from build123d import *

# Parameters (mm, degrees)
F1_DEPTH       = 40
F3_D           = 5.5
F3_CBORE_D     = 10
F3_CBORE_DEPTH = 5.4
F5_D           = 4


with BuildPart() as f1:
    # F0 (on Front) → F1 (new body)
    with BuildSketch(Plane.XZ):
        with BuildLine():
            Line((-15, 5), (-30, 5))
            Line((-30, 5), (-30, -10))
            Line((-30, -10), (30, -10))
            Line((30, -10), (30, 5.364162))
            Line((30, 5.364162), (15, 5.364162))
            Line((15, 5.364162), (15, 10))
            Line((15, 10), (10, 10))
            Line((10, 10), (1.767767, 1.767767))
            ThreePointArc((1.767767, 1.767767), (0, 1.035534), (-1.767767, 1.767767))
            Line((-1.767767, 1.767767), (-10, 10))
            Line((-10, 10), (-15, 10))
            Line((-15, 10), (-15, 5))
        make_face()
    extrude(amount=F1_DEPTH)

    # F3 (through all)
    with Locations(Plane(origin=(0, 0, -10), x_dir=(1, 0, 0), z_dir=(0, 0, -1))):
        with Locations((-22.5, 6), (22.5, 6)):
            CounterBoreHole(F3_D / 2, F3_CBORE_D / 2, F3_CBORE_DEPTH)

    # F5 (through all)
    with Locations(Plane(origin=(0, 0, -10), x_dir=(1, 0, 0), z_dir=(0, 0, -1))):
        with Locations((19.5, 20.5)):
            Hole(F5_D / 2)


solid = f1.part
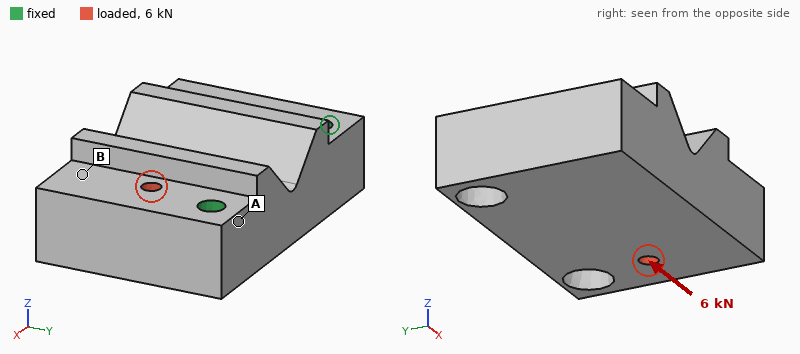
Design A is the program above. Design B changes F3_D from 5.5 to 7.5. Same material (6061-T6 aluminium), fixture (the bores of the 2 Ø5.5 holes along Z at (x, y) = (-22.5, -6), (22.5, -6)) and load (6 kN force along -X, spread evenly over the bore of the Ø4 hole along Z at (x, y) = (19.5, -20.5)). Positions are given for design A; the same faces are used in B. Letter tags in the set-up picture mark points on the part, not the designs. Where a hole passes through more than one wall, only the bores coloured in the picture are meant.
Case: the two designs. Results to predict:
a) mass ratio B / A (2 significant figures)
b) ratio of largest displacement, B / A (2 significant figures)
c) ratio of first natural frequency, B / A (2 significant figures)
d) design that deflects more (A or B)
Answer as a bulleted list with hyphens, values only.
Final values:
- 0.99
- 0.90
- 1.2
- A
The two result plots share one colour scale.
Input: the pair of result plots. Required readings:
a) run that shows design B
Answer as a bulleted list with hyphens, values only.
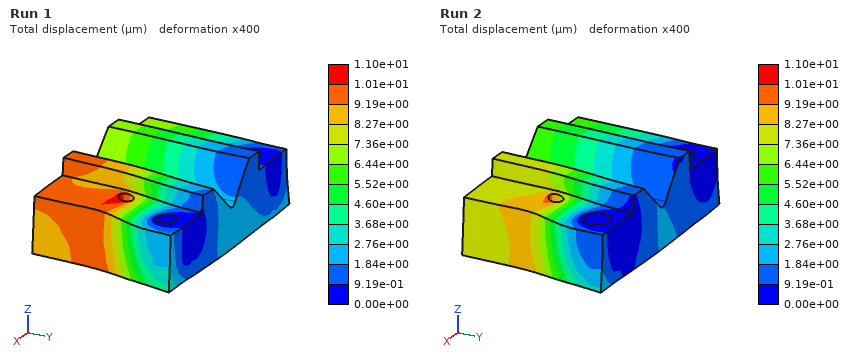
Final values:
- Run 2
